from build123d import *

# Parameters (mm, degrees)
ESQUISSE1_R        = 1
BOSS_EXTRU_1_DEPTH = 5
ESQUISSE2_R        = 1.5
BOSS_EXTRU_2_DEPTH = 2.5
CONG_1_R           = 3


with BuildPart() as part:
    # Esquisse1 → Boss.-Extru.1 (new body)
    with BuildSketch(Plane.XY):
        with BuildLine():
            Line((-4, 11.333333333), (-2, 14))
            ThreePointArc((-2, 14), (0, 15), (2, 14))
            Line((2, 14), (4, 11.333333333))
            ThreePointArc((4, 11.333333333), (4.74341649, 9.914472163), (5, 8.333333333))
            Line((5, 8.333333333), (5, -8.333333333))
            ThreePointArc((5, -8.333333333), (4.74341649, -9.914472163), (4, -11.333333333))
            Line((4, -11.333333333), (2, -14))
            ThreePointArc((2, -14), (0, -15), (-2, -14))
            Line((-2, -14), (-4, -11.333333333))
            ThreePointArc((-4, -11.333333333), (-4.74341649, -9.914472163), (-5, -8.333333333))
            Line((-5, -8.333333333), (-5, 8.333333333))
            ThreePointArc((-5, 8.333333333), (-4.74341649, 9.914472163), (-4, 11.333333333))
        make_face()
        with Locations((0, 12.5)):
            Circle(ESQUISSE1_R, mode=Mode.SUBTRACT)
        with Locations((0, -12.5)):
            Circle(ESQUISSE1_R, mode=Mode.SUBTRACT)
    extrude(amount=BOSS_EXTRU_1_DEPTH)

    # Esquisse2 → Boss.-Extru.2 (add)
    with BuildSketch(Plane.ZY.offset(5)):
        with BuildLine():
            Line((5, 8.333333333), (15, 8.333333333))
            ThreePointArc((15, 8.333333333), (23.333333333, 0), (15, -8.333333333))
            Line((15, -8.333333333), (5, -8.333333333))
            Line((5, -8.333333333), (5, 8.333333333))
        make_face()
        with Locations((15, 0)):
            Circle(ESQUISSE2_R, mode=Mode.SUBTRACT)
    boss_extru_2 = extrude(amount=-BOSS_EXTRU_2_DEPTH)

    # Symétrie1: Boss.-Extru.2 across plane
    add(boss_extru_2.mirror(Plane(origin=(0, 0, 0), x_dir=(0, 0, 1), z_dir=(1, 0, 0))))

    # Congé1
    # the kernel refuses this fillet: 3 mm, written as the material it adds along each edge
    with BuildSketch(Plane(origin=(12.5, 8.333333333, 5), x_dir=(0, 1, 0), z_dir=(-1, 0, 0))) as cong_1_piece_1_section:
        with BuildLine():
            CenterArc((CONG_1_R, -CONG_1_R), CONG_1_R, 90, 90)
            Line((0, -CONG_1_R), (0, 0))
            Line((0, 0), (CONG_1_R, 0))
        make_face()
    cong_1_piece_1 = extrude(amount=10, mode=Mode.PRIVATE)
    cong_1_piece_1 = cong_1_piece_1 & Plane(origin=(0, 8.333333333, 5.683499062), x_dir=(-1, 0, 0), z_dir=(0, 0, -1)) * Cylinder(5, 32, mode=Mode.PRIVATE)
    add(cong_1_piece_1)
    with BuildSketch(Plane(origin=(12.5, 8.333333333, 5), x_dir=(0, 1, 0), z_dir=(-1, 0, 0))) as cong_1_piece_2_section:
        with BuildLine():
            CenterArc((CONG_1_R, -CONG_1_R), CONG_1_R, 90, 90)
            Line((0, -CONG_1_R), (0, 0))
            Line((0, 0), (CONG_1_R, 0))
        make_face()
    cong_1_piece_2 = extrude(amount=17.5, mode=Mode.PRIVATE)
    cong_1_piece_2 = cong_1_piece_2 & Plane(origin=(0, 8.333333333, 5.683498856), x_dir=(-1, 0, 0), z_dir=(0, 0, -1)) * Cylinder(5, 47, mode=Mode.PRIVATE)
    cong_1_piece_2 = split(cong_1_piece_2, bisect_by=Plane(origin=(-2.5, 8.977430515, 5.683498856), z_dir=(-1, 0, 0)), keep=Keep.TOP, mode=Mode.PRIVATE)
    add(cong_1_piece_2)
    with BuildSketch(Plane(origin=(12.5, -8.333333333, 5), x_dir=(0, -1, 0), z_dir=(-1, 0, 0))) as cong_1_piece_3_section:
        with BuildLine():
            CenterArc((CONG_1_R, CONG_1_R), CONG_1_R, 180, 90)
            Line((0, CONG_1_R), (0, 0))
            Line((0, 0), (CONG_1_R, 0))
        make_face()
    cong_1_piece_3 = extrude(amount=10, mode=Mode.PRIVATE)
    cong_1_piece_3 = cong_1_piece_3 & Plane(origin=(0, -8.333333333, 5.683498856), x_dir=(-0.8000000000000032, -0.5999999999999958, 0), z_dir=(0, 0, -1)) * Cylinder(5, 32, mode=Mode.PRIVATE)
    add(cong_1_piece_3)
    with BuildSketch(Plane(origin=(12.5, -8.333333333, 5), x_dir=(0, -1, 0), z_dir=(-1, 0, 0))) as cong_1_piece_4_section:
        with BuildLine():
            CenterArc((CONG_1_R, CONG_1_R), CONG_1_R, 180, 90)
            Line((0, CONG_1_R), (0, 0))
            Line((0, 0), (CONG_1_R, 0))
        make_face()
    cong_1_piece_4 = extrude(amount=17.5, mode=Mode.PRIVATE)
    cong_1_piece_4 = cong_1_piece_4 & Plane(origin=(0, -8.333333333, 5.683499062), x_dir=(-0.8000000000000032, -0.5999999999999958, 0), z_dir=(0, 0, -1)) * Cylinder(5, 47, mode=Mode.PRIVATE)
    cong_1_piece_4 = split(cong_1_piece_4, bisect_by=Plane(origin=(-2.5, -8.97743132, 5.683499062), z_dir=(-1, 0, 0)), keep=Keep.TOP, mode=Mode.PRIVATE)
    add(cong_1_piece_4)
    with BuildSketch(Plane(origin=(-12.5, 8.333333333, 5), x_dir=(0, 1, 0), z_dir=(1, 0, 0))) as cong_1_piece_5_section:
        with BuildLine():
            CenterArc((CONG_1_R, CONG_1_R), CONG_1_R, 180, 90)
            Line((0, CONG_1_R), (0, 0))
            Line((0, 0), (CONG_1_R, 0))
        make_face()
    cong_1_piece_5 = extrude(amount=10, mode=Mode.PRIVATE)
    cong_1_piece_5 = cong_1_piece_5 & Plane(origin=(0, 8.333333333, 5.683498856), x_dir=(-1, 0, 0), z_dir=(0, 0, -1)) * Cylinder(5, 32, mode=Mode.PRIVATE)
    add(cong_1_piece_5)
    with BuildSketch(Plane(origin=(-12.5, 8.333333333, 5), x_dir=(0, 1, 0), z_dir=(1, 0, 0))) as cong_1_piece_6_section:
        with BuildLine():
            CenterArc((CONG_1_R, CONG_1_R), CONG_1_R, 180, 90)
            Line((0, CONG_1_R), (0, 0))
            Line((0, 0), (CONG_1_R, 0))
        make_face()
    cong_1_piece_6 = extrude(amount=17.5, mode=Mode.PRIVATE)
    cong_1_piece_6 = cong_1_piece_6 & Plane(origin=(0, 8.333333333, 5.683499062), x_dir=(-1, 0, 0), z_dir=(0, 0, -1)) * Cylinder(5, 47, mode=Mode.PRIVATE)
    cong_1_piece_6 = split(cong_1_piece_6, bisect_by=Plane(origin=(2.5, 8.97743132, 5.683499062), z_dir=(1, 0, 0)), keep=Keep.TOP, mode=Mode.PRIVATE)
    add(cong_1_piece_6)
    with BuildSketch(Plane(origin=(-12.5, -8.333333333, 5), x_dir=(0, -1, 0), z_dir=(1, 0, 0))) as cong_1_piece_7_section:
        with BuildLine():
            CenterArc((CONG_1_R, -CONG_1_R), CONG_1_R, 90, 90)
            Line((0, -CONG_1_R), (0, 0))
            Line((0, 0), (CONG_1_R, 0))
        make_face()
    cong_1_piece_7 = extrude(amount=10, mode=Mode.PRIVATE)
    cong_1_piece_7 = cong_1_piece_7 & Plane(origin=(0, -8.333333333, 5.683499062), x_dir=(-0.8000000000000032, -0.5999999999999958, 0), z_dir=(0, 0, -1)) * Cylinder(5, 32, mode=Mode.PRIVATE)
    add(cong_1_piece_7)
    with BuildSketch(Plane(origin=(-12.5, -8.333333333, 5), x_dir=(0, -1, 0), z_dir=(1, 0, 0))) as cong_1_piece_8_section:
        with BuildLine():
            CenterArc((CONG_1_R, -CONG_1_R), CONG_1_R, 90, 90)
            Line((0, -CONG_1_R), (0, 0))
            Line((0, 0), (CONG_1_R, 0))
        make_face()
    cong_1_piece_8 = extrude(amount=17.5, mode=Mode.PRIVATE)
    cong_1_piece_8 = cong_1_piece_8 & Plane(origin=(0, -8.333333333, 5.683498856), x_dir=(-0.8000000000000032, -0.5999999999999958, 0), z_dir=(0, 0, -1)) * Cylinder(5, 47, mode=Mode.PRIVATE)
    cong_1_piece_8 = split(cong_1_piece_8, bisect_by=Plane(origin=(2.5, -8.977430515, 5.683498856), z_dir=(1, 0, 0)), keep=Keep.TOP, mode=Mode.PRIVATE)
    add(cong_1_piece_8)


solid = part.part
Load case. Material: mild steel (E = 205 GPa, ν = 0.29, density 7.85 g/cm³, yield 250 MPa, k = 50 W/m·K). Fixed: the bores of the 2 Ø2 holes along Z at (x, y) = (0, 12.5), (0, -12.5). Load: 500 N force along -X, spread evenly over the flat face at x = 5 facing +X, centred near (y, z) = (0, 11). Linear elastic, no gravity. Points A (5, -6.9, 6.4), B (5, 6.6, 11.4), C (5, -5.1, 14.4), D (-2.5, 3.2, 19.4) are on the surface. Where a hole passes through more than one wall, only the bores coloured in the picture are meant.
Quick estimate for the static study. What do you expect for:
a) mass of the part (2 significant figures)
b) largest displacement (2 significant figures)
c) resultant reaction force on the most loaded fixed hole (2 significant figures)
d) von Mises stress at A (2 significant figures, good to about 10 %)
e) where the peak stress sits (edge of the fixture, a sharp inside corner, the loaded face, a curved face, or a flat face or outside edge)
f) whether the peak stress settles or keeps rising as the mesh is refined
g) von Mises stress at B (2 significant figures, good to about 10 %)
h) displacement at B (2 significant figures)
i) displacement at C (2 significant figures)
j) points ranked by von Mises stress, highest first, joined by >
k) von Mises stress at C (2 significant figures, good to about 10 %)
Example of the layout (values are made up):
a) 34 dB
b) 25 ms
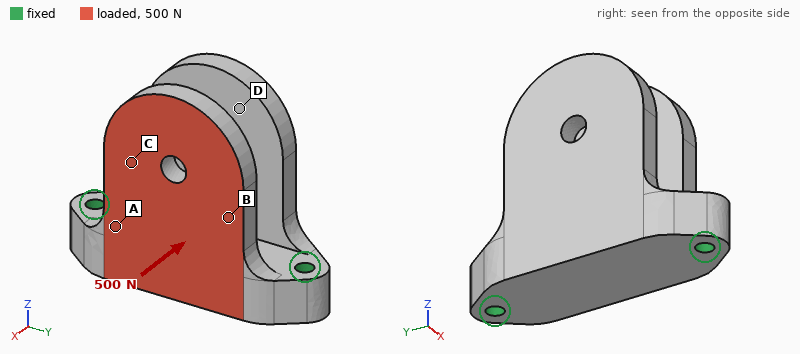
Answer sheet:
a) 21 g
b) 90 µm
c) 250 N
d) 150 MPa
e) edge of the fixture
f) keeps rising
g) 78 MPa
h) 26 µm
i) 40 µm
j) A > B > C > D
k) 45 MPa
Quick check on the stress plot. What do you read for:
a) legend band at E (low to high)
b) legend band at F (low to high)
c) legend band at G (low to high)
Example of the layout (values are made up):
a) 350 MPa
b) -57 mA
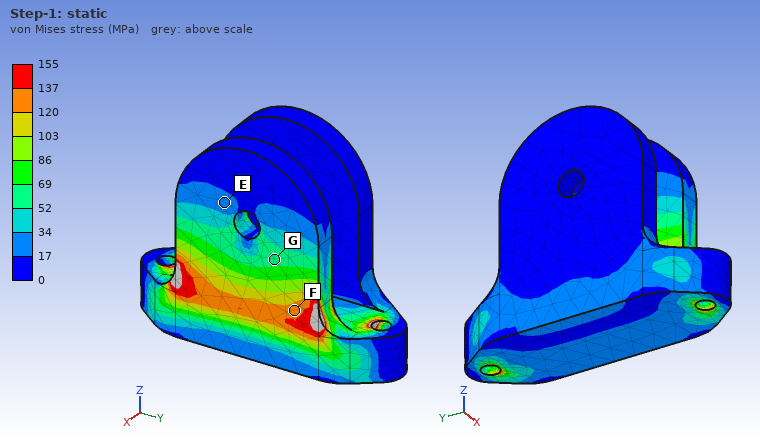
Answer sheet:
a) 17 to 34 MPa
b) 120 to 137 MPa
c) 52 to 69 MPa
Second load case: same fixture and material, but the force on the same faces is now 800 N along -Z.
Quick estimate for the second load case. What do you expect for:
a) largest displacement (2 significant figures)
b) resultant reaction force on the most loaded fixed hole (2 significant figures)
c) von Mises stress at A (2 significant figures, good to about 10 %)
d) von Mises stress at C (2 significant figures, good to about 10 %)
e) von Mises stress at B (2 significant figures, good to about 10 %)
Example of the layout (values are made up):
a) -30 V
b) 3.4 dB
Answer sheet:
a) 38 µm
b) 420 N
c) 60 MPa
d) 29 MPa
e) 41 MPa
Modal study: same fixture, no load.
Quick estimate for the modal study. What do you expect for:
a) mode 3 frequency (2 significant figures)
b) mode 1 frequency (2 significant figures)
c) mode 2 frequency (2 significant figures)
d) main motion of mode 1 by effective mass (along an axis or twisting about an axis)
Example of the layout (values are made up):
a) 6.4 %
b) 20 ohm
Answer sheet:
a) 17 kHz
b) 5500 Hz
c) 6400 Hz
d) along X
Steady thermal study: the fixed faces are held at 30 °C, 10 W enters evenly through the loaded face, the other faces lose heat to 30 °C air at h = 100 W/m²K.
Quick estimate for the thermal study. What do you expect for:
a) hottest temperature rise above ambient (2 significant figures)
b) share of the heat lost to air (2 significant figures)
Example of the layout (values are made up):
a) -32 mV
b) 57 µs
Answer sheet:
a) 43 K
b) 24 %
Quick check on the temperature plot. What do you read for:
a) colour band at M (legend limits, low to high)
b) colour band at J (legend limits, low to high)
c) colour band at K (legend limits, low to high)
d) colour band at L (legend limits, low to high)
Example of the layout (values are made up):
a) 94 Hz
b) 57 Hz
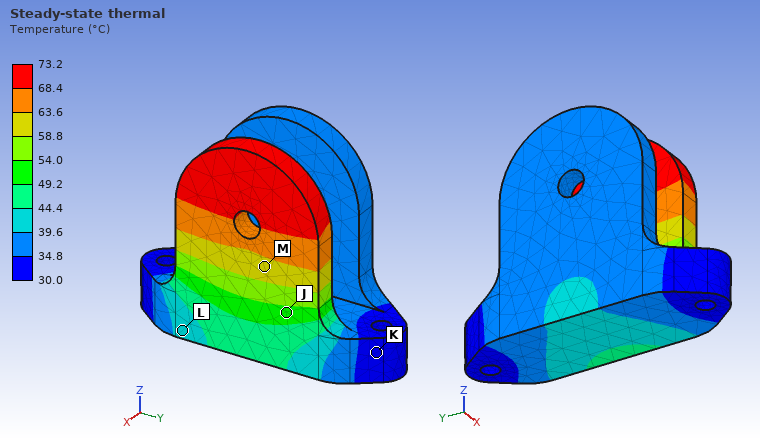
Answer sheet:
a) 58.8 to 63.6 °C
b) 49.2 to 54.0 °C
c) 30.0 to 34.8 °C
d) 39.6 to 44.4 °C
